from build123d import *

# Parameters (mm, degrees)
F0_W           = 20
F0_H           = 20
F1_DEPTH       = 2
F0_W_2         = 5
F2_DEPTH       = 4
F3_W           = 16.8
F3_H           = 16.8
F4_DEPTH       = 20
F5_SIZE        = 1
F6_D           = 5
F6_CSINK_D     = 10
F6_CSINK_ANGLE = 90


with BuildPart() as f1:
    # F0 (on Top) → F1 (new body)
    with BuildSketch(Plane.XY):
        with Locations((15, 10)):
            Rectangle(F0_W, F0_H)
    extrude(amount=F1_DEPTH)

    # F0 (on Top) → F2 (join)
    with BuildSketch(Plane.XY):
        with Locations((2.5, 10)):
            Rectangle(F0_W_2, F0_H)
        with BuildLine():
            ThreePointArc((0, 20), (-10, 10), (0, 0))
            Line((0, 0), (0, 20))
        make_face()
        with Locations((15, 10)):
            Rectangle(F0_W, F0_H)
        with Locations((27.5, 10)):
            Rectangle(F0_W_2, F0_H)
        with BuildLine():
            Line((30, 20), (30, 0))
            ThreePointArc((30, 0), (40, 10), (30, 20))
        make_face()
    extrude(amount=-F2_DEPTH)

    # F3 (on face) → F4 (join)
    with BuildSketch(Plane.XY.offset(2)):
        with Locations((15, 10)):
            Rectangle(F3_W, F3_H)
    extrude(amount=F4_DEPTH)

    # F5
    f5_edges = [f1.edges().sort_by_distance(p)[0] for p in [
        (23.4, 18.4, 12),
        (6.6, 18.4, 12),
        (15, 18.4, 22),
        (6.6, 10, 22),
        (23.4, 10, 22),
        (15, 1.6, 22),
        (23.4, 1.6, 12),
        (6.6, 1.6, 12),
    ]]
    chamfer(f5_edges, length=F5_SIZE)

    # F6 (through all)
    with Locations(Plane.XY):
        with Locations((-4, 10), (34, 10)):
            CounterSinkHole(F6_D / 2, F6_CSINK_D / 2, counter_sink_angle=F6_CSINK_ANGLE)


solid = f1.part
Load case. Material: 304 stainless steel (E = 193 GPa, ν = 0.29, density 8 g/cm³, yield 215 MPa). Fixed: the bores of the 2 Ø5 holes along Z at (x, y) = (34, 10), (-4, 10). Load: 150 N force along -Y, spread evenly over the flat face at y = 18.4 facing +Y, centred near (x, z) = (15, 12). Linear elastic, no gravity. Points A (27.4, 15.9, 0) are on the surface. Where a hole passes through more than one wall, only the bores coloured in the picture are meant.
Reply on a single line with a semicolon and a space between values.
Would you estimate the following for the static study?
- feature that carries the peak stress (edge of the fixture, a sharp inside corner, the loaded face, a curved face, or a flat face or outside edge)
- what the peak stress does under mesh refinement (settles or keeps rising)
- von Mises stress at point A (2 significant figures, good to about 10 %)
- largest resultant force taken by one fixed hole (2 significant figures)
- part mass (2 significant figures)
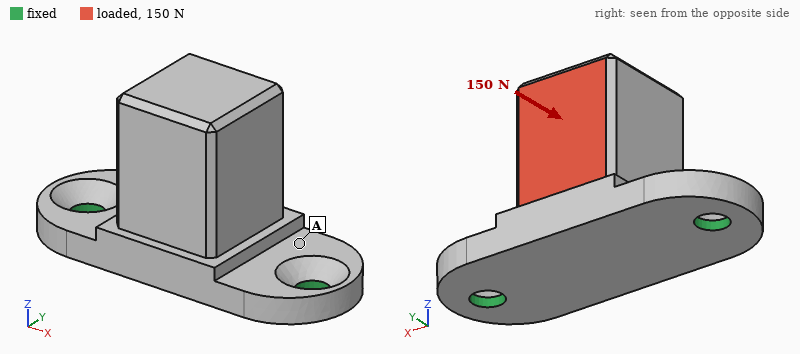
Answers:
edge of the fixture; keeps rising; 12 MPa; 75 N; 78 g
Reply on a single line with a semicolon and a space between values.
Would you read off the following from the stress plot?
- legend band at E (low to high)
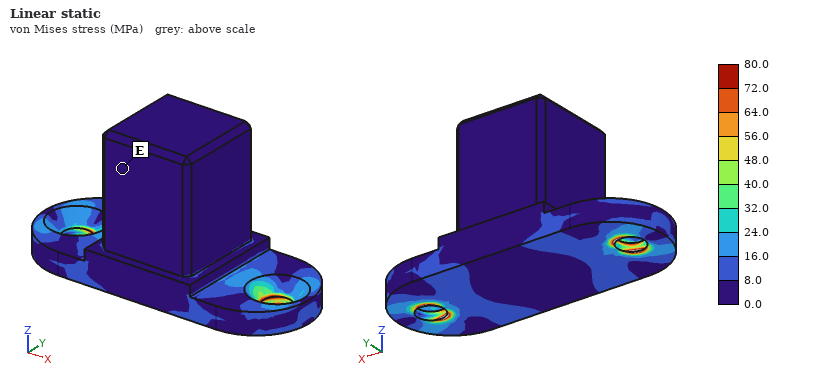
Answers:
0.0 to 8.0 MPa
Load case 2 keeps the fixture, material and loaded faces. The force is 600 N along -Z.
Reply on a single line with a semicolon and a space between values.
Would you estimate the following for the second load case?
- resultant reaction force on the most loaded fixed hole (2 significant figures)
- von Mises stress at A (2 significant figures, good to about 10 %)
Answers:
470 N; 35 MPa
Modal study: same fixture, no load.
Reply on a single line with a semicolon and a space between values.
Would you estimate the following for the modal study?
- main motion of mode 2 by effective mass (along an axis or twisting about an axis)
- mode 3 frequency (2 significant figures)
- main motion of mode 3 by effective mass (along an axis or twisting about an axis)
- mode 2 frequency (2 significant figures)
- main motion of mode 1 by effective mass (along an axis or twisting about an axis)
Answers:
along Z; 8500 Hz; along X; 8000 Hz; along Y
